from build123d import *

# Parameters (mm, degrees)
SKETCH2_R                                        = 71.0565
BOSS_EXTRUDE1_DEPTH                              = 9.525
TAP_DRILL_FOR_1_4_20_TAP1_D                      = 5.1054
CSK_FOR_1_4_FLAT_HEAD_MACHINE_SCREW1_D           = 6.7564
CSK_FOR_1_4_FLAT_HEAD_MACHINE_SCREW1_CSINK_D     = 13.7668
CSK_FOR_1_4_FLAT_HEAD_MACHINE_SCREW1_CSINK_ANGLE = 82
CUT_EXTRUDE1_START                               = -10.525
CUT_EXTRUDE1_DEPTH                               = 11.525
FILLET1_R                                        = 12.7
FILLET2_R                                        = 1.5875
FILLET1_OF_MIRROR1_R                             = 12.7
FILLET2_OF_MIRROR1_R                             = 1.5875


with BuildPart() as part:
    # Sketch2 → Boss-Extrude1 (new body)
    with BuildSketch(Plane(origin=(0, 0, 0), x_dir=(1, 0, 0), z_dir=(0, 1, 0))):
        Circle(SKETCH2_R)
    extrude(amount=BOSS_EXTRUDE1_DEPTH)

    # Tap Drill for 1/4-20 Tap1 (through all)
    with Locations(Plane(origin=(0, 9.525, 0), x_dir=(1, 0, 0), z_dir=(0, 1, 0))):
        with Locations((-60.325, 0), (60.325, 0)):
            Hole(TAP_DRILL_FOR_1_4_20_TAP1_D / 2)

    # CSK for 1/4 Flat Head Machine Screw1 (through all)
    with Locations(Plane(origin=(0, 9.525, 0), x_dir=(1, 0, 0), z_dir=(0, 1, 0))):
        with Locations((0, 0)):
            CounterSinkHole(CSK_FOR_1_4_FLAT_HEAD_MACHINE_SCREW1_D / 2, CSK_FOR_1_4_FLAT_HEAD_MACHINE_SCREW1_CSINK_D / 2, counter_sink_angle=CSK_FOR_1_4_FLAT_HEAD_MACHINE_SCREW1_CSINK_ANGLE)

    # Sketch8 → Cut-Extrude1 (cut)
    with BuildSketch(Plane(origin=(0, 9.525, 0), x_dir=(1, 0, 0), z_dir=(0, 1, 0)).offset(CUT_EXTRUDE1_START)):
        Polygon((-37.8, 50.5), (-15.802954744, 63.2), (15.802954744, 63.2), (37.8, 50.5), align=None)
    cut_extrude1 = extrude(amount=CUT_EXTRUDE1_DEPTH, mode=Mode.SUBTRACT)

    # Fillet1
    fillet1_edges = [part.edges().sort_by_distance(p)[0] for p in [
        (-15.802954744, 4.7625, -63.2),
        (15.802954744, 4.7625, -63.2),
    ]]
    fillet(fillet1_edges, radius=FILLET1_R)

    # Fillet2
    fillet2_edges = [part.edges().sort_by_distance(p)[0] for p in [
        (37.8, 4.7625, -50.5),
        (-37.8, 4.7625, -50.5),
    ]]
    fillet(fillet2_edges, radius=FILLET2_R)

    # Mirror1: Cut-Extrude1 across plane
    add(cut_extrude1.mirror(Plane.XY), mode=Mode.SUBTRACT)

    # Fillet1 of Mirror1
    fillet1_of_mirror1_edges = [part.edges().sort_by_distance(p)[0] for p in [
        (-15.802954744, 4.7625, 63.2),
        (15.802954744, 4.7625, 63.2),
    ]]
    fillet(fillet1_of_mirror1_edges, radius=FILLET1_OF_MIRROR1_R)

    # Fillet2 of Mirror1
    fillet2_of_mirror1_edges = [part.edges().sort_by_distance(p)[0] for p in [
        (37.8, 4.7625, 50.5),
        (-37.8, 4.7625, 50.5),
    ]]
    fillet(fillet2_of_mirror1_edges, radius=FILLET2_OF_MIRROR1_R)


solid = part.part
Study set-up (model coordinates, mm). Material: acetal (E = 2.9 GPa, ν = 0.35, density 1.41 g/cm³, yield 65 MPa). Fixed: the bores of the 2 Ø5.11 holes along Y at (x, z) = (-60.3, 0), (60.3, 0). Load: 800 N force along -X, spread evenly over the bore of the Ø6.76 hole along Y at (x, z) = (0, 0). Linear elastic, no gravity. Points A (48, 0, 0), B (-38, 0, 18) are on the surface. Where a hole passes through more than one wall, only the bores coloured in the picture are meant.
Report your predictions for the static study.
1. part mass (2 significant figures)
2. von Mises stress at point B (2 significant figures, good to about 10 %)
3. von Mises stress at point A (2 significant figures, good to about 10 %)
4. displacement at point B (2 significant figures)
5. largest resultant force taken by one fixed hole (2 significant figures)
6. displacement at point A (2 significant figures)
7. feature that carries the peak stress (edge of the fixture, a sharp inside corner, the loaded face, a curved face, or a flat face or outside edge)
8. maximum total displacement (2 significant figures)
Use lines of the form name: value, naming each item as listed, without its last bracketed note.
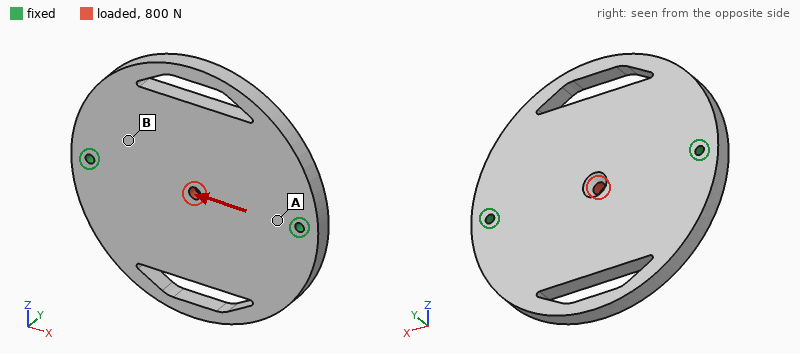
part mass: 190 g
von Mises stress at point B: 0.77 MPa
von Mises stress at point A: 1.8 MPa
displacement at point B: 15 µm
largest resultant force taken by one fixed hole: 400 N
displacement at point A: 7.7 µm
feature that carries the peak stress: the loaded face
maximum total displacement: 45 µm
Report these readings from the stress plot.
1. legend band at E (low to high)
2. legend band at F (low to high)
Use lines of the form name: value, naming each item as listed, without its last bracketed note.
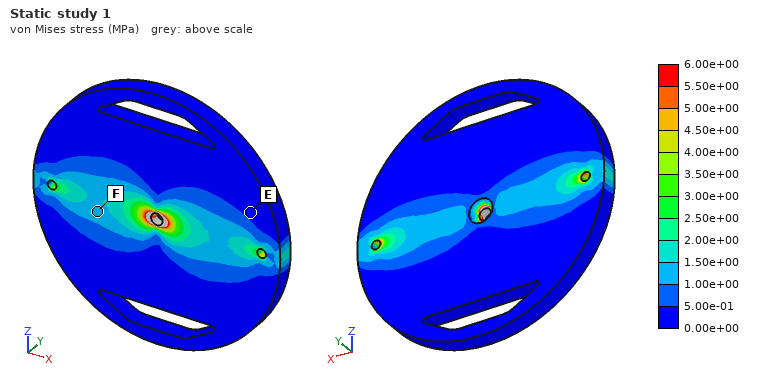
legend band at E: 0.00e+00 to 5.00e-01 MPa
legend band at F: 1.00e+00 to 1.50e+00 MPa
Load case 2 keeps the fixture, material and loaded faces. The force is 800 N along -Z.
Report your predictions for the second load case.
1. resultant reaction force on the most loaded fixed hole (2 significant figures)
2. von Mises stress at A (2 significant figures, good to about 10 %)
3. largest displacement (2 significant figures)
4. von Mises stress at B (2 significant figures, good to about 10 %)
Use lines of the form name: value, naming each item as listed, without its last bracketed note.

resultant reaction force on the most loaded fixed hole: 400 N
von Mises stress at A: 1.6 MPa
largest displacement: 0.13 mm
von Mises stress at B: 1.2 MPa
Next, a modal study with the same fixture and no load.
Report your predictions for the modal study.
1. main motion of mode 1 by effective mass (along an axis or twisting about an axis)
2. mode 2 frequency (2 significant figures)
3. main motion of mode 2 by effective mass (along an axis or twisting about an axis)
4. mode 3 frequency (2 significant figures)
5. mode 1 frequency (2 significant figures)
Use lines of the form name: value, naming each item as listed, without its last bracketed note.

main motion of mode 1 by effective mass: twisting about X
mode 2 frequency: 480 Hz
main motion of mode 2 by effective mass: along Y
mode 3 frequency: 950 Hz
mode 1 frequency: 340 Hz
